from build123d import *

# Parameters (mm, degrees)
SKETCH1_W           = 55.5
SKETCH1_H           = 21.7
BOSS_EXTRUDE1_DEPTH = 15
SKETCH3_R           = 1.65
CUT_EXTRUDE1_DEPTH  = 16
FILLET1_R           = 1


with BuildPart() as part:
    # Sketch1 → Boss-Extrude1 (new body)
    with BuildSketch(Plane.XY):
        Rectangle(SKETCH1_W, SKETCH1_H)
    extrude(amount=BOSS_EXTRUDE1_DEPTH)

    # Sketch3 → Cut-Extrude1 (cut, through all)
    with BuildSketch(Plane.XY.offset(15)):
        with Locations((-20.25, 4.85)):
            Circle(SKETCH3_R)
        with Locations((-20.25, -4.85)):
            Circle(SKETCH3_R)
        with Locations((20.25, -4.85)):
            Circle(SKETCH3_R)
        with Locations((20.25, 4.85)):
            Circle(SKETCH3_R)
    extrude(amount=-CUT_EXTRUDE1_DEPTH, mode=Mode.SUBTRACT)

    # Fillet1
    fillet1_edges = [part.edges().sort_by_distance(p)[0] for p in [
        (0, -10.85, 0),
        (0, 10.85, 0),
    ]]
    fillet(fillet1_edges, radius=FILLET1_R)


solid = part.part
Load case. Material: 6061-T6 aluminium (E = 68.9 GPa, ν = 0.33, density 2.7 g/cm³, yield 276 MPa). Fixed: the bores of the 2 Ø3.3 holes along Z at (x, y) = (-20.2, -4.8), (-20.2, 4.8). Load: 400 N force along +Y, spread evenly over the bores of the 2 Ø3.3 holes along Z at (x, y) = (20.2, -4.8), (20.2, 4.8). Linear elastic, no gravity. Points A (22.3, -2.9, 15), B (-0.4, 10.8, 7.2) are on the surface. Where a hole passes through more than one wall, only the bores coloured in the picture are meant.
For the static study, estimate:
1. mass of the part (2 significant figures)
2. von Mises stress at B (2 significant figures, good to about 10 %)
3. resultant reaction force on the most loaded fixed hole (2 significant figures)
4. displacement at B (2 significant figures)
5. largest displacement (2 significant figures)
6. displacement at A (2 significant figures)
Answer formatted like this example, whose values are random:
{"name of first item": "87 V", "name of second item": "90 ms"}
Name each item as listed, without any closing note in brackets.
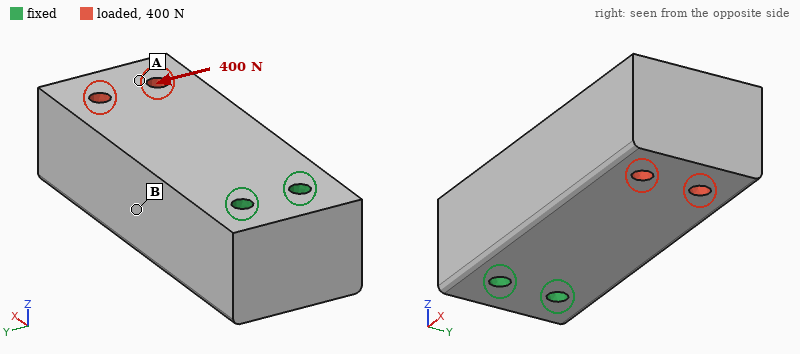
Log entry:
{"mass of the part": "47 g", "von Mises stress at B": "7.1 MPa", "resultant reaction force on the most loaded fixed hole": "1.4 kN", "displacement at B": "6.5 µm", "largest displacement": "18 µm", "displacement at A": "16 µm"}
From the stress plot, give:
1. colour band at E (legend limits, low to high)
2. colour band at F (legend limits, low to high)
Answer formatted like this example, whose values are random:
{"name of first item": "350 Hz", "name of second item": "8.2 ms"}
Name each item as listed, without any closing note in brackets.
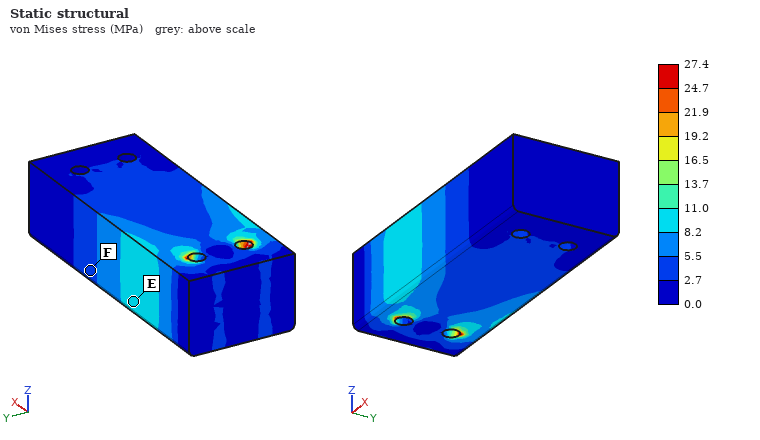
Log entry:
{"colour band at E": "8.2 to 11.0 MPa", "colour band at F": "2.7 to 5.5 MPa"}
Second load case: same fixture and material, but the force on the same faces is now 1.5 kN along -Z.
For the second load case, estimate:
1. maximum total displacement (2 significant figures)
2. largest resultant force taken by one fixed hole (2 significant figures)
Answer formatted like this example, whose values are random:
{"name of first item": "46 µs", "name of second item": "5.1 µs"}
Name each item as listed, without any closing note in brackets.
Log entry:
{"maximum total displacement": "0.11 mm", "largest resultant force taken by one fixed hole": "750 N"}
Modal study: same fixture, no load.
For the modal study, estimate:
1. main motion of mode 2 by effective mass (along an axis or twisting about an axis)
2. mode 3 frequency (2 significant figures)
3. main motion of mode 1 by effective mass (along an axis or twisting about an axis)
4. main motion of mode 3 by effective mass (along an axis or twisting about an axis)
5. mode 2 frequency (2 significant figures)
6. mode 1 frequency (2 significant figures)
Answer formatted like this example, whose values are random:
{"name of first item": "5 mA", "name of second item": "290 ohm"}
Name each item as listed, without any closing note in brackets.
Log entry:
{"main motion of mode 2 by effective mass": "along Y", "mode 3 frequency": "14 kHz", "main motion of mode 1 by effective mass": "along Z", "main motion of mode 3 by effective mass": "twisting about X", "mode 2 frequency": "6200 Hz", "mode 1 frequency": "5000 Hz"}
